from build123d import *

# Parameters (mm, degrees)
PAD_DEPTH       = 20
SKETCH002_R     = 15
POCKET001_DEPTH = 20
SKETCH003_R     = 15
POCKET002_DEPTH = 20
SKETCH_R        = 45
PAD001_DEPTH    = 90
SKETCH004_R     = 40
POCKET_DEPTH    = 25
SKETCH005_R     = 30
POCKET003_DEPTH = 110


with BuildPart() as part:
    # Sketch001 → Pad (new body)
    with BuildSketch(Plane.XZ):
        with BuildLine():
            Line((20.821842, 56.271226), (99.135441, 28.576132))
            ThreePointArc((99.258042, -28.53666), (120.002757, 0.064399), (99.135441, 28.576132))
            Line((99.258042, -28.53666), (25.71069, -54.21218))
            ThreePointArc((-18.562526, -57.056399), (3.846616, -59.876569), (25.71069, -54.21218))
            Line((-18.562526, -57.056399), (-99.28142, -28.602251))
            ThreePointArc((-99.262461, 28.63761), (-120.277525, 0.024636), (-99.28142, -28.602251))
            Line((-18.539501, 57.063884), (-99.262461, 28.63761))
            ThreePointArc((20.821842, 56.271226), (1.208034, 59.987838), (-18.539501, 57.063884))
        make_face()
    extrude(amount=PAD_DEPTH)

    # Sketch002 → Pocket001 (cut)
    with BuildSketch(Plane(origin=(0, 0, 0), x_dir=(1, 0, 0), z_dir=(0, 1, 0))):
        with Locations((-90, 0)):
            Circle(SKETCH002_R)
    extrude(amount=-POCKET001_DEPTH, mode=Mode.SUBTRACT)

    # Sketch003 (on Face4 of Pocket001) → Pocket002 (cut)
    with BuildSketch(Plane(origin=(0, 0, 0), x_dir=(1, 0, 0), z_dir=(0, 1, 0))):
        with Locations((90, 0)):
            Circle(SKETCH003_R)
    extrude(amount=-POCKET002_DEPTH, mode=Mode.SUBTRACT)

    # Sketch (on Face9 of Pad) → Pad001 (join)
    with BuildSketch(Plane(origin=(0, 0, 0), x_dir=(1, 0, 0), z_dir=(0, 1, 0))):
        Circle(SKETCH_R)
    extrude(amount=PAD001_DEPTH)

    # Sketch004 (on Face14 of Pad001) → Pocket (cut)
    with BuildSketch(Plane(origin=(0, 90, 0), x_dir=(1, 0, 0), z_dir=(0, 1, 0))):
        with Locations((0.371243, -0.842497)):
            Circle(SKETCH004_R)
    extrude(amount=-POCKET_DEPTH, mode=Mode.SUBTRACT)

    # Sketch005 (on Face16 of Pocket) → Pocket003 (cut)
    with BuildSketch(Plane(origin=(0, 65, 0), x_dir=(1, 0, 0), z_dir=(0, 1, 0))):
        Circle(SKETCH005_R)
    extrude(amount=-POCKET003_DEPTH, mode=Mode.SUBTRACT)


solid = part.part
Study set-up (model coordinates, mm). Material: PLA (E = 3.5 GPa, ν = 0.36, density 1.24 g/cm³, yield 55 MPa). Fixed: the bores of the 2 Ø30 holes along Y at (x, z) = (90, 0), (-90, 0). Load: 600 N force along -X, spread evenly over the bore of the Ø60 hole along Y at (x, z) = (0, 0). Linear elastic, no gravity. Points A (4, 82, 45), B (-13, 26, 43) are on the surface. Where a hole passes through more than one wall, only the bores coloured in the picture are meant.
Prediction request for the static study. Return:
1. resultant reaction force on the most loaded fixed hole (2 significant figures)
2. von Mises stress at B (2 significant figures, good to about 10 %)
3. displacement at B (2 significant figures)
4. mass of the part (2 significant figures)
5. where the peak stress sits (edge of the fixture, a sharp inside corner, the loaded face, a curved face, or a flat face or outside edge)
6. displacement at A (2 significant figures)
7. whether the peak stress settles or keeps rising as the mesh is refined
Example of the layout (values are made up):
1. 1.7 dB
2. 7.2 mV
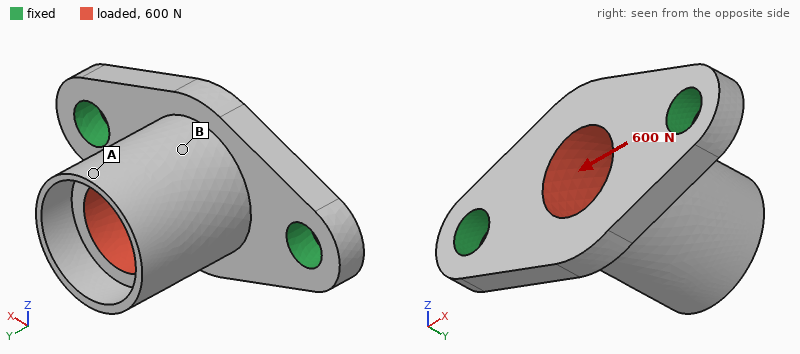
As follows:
1. 340 N
2. 0.17 MPa
3. 13 µm
4. 720 g
5. edge of the fixture
6. 28 µm
7. keeps rising
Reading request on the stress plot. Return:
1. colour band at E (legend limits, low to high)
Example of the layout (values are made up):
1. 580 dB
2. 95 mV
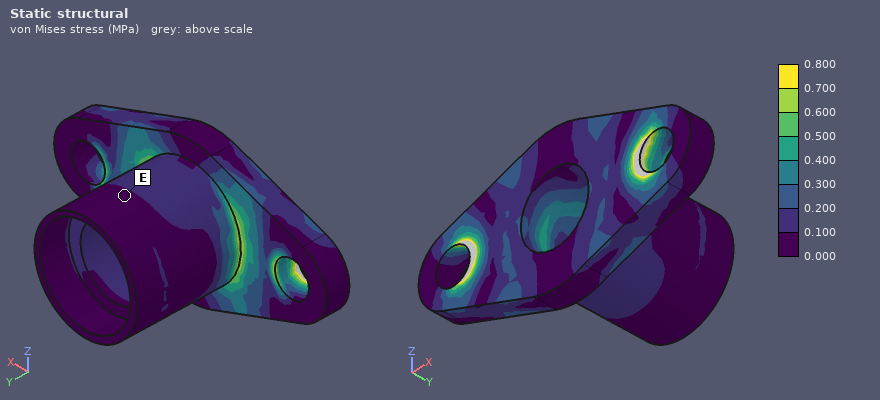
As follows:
1. 0.000 to 0.100 MPa
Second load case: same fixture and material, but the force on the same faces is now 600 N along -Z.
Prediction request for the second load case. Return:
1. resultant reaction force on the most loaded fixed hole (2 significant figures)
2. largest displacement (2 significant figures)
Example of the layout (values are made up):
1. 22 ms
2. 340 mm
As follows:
1. 300 N
2. 0.18 mm
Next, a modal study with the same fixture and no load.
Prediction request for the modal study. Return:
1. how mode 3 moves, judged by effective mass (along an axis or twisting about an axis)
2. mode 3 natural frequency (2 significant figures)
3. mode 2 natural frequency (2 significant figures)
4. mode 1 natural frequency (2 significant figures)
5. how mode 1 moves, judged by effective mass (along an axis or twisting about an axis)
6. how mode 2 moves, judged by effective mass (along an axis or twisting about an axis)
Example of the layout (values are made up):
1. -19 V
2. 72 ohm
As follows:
1. along X
2. 1100 Hz
3. 940 Hz
4. 470 Hz
5. along Z
6. along Y
